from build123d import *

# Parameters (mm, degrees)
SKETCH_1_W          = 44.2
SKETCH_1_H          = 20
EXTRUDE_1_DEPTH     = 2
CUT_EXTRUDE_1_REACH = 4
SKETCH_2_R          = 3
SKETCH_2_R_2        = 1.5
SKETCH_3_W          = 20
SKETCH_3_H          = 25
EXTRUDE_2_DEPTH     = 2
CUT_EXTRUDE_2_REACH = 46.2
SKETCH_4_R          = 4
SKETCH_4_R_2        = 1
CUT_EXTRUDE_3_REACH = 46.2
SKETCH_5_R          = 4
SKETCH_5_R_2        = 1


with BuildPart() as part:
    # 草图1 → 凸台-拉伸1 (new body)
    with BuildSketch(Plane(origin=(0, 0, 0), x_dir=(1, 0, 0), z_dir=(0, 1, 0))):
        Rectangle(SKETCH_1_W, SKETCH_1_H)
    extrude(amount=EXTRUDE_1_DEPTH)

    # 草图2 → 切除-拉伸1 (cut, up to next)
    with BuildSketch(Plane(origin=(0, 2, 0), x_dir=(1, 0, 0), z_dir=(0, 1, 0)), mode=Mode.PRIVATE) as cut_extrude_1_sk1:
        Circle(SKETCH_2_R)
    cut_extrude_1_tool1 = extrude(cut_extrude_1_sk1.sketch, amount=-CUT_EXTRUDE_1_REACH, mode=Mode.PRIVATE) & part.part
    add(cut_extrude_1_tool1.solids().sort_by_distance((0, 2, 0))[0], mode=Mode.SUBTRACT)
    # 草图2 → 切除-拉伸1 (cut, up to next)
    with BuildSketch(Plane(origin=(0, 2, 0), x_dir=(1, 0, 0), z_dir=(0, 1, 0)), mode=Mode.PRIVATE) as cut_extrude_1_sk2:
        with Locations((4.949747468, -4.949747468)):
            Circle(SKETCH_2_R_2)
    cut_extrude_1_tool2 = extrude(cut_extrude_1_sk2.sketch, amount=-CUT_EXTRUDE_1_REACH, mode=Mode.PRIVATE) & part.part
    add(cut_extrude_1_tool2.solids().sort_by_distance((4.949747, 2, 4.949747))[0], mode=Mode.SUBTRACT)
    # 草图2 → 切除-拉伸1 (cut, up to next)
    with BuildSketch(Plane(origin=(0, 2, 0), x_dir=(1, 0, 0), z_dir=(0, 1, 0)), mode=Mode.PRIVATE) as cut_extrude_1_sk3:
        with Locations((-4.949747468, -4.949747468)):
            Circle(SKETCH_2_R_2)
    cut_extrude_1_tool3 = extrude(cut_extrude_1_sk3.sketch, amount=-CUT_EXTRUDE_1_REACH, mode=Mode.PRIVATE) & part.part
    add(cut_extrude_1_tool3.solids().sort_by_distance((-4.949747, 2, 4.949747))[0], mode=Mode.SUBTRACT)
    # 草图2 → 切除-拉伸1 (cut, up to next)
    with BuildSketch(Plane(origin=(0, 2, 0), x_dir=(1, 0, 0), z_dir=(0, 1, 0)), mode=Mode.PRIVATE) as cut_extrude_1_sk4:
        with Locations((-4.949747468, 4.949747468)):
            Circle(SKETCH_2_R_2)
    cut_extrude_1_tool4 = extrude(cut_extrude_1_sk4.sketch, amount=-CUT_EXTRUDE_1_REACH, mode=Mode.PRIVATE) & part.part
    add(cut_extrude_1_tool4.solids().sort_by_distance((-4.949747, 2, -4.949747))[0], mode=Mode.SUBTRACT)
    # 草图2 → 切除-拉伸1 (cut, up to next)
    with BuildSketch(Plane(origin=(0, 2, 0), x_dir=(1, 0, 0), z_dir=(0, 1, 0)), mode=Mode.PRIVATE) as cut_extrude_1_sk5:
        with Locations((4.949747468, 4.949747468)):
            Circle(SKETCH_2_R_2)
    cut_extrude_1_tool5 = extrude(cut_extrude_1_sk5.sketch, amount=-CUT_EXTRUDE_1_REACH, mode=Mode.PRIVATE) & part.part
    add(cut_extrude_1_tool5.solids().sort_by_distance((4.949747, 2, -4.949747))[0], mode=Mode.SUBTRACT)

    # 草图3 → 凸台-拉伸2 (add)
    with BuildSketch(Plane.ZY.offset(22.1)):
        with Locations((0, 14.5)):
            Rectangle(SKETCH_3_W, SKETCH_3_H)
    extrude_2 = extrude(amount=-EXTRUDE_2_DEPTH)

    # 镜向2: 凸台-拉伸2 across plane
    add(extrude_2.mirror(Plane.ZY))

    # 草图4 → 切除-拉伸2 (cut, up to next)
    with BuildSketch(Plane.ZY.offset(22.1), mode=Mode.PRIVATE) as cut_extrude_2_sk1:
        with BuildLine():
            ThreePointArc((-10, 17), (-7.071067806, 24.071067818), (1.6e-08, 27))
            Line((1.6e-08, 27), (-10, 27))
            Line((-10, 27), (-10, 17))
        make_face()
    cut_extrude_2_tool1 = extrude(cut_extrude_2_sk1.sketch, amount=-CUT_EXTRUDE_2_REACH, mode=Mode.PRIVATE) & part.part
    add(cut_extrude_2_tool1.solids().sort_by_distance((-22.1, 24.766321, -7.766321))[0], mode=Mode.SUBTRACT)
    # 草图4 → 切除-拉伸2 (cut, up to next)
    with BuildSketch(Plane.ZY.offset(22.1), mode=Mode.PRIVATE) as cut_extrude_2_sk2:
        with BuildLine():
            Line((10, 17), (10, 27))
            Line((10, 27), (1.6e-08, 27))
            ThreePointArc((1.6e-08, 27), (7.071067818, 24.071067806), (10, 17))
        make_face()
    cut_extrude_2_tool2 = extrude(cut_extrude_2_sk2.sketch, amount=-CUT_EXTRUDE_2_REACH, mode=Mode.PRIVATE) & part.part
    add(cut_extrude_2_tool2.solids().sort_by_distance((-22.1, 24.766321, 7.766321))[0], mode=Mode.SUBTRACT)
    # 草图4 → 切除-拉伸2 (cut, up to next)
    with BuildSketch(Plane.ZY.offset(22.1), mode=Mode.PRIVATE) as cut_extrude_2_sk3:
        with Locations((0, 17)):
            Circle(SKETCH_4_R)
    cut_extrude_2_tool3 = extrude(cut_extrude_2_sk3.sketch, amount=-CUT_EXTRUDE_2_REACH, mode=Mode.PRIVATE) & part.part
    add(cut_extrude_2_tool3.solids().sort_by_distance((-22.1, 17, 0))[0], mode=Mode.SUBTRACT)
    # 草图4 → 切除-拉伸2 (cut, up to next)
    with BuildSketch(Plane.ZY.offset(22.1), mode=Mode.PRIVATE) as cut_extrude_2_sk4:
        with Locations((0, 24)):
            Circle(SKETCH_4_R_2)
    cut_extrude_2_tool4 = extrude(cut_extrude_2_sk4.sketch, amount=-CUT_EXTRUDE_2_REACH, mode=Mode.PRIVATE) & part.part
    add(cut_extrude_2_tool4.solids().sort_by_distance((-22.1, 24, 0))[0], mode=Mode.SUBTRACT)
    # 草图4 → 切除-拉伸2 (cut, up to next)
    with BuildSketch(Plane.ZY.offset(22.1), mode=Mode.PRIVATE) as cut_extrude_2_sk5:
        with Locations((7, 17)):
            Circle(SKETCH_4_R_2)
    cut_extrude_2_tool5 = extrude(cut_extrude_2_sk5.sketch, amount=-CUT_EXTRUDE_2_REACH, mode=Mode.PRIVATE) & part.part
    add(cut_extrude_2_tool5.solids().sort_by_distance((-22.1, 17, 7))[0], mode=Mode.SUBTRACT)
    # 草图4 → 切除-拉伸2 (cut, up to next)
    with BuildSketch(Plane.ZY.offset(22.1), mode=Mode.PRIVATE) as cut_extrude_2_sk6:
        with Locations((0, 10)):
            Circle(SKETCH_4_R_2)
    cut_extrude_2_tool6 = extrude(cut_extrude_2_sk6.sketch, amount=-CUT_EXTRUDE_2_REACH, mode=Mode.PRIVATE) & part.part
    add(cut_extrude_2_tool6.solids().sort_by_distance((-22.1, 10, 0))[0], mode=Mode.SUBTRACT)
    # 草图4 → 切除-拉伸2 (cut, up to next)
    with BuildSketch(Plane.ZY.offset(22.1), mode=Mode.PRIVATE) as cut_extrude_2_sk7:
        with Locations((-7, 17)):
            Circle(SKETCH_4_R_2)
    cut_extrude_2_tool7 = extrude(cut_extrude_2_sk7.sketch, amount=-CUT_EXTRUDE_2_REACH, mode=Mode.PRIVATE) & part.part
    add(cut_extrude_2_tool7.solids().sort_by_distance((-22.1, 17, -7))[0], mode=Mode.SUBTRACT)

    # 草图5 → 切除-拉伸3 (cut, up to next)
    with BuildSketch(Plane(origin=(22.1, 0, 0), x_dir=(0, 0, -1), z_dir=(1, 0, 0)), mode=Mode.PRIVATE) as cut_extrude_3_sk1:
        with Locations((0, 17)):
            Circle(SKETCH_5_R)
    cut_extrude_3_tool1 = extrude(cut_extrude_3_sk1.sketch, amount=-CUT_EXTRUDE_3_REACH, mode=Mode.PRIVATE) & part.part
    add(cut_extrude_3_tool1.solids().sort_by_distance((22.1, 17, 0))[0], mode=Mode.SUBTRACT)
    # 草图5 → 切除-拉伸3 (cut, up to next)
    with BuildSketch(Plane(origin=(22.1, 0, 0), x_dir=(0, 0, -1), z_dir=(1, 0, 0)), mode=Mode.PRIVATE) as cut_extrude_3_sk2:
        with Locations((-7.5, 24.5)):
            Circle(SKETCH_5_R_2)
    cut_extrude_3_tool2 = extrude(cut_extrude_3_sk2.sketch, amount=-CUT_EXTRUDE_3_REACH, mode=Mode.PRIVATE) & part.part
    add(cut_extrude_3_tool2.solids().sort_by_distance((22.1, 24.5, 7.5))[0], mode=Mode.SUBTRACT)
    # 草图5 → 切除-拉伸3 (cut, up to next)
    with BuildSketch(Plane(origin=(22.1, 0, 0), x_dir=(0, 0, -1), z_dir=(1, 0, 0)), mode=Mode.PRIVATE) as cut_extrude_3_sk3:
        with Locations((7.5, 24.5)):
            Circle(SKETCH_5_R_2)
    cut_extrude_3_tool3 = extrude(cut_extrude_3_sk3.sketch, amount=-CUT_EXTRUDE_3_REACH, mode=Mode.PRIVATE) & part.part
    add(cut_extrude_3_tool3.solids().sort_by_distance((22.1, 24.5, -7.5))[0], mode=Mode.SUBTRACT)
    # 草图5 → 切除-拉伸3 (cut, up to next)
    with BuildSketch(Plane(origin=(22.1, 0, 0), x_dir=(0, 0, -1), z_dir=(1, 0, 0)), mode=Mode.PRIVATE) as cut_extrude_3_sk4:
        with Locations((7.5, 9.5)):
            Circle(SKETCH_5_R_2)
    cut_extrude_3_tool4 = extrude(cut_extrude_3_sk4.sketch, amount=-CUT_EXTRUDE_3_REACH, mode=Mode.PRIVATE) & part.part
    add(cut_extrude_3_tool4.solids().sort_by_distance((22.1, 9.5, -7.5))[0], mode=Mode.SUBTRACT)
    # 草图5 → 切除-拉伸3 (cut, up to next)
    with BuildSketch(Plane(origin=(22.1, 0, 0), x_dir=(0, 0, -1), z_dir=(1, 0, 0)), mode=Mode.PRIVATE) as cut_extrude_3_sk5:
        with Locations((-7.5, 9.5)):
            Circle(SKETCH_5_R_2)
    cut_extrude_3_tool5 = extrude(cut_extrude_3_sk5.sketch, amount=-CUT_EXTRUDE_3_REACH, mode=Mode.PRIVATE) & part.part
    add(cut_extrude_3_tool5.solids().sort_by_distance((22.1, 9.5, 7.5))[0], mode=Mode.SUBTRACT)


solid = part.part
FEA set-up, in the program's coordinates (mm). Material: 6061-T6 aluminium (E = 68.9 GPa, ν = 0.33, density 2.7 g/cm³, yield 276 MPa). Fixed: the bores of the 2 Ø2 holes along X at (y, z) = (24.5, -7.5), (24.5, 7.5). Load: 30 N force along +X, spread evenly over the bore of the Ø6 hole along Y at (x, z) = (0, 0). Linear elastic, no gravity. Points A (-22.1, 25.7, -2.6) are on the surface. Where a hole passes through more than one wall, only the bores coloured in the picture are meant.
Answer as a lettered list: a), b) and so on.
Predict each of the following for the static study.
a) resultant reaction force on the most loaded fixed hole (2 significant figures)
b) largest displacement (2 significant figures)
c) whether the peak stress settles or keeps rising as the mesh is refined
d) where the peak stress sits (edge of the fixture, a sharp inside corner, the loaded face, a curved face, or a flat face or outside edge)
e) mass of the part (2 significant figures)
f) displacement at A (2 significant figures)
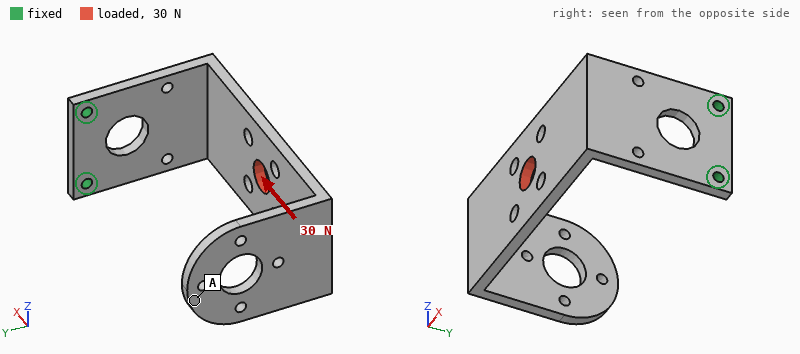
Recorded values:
a) 15 N
b) 0.56 mm
c) keeps rising
d) edge of the fixture
e) 9.0 g
f) 0.54 mm
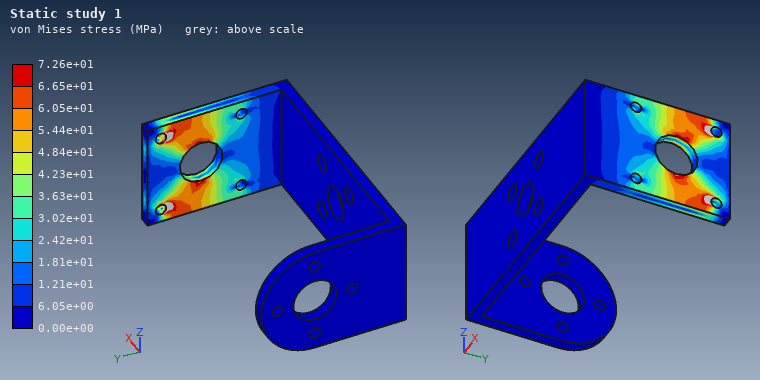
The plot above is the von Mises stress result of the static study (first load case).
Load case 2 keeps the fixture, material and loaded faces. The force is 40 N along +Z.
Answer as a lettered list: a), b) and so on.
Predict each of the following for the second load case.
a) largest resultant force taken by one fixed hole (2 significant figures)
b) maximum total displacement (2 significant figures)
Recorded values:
a) 79 N
b) 0.57 mm
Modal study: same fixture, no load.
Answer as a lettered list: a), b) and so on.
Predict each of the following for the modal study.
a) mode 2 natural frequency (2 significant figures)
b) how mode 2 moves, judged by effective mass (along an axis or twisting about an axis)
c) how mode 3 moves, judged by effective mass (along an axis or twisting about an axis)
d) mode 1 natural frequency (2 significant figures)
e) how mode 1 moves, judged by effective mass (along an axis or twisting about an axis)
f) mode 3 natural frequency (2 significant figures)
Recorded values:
a) 480 Hz
b) along Z
c) along X
d) 280 Hz
e) along Y
f) 910 Hz
